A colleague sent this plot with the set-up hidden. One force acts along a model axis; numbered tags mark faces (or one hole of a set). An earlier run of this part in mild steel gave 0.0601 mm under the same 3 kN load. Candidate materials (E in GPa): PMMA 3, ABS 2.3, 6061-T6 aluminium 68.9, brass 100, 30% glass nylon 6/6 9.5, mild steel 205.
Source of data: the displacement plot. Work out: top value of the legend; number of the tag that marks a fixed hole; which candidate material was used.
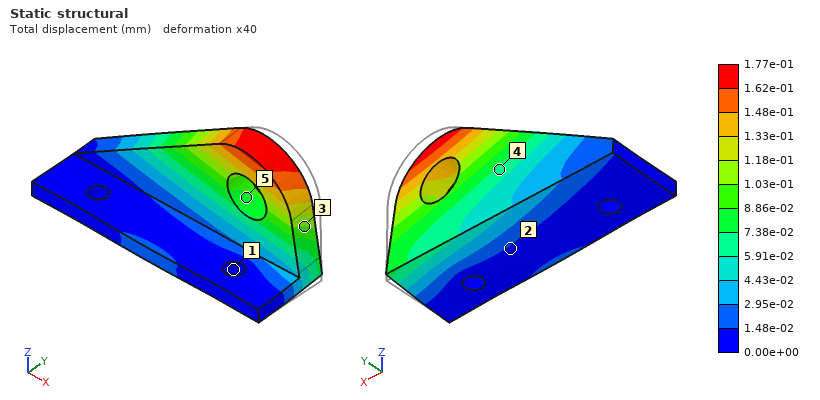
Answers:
1.77e-01 mm
1
6061-T6 aluminium
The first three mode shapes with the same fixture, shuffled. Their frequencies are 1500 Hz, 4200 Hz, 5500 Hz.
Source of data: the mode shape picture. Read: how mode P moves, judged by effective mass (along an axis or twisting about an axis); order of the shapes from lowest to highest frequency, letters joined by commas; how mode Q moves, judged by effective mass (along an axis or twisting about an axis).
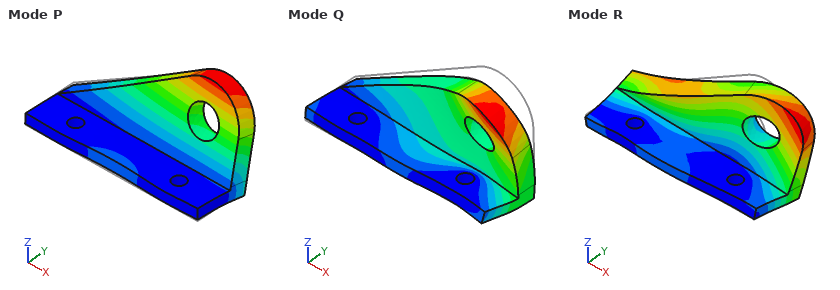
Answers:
along Y
P, R, Q
along Z
